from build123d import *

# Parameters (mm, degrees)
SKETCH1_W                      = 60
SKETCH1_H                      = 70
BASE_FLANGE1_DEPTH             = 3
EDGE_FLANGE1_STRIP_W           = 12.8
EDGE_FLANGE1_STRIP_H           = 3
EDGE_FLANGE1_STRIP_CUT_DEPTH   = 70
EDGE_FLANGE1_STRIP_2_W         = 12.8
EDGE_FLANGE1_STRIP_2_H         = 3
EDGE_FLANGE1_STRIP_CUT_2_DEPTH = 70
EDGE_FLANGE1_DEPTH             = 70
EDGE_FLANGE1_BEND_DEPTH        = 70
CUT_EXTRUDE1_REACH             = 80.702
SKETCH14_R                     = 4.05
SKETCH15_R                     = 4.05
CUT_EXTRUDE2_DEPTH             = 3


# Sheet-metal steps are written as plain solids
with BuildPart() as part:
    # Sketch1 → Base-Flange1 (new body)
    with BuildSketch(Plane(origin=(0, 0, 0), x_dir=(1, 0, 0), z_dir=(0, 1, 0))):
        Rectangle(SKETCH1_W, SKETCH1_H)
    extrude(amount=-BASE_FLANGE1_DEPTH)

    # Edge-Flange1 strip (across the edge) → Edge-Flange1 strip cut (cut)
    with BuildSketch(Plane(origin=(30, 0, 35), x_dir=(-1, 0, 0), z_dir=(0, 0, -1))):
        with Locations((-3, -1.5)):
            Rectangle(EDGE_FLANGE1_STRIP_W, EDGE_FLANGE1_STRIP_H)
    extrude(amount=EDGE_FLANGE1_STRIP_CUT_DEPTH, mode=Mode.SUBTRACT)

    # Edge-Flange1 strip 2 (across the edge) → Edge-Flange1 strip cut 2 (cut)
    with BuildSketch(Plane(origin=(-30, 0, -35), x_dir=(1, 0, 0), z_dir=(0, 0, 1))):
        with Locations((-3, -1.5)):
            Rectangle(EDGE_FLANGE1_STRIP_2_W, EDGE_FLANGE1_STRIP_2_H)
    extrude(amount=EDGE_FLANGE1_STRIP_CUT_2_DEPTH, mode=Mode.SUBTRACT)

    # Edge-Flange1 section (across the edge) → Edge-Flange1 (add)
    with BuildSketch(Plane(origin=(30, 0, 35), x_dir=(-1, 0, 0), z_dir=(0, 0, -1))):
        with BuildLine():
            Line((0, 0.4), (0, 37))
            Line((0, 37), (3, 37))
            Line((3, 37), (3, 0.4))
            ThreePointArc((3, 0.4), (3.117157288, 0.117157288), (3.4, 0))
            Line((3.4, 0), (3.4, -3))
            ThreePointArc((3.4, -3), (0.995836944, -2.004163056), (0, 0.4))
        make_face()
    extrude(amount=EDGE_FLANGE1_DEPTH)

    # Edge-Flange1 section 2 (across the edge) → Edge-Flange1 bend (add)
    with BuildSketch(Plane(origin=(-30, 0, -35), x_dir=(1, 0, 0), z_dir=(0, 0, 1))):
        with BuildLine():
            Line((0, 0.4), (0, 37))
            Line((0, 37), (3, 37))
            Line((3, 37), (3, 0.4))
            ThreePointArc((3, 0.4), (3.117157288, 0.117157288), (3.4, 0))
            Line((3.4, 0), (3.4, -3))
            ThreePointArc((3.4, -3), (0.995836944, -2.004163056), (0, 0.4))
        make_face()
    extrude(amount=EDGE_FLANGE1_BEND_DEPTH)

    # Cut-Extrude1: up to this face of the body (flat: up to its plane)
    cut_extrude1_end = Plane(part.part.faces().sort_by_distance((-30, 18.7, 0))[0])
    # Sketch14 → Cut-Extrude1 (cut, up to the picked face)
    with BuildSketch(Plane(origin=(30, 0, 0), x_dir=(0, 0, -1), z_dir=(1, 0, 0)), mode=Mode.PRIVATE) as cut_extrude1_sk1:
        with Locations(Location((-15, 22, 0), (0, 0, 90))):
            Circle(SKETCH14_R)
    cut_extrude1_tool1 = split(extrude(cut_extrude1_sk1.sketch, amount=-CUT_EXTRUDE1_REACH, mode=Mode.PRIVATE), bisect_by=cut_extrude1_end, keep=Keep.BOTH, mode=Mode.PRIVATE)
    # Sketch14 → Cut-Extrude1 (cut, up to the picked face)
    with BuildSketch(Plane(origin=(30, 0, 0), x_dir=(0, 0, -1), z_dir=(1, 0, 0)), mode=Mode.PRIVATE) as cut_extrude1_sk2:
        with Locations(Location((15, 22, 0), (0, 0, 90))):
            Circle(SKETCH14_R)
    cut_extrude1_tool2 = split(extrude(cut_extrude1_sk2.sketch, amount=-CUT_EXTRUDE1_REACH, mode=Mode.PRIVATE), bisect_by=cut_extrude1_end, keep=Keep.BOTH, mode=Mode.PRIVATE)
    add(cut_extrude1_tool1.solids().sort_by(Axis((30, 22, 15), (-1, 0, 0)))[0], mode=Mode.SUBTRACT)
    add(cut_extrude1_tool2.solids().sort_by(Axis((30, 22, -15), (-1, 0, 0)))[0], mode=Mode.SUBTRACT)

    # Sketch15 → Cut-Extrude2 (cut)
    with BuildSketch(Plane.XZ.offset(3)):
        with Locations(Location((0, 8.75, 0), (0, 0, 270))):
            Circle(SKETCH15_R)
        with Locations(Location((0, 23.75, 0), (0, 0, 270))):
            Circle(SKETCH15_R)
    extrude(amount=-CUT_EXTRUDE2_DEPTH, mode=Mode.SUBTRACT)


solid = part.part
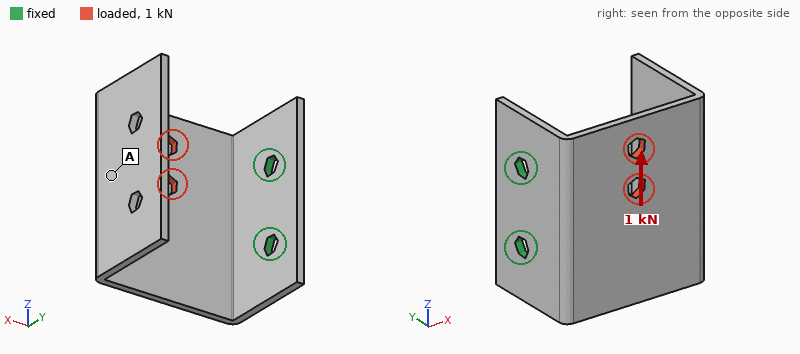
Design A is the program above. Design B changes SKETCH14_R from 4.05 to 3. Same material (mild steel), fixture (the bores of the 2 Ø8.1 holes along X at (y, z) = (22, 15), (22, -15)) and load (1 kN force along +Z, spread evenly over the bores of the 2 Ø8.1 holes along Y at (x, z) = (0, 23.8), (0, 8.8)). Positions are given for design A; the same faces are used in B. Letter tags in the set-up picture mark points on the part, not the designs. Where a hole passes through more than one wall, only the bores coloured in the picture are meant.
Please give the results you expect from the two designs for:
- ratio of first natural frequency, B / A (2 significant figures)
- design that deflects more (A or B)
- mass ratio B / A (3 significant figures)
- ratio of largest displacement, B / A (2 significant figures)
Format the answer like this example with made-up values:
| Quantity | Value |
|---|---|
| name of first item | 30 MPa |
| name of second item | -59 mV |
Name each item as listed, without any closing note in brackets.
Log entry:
| Quantity | Value |
|---|---|
| ratio of first natural frequency, B / A | 0.98 |
| design that deflects more | B |
| mass ratio B / A | 1.01 |
| ratio of largest displacement, B / A | 1.1 |
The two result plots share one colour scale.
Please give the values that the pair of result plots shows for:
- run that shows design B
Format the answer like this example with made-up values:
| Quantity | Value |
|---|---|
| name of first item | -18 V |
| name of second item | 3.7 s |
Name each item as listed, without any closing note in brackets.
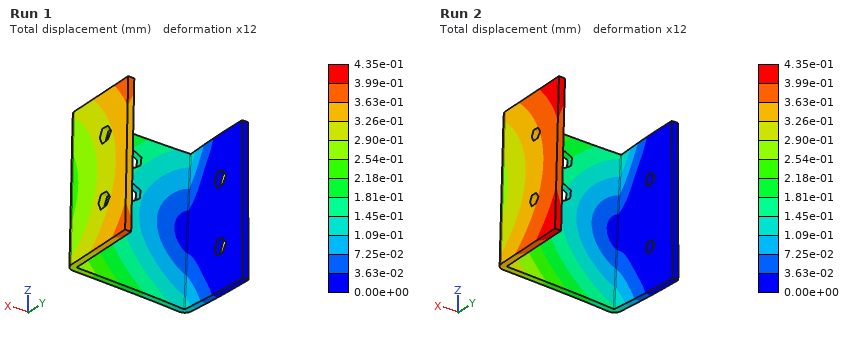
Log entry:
| Quantity | Value |
|---|---|
| run that shows design B | Run 2 |
